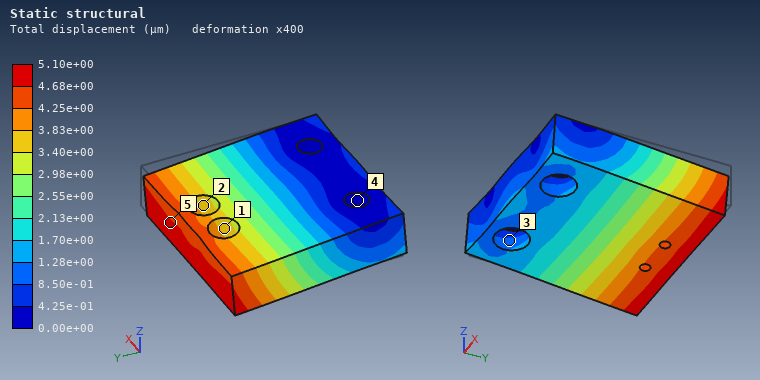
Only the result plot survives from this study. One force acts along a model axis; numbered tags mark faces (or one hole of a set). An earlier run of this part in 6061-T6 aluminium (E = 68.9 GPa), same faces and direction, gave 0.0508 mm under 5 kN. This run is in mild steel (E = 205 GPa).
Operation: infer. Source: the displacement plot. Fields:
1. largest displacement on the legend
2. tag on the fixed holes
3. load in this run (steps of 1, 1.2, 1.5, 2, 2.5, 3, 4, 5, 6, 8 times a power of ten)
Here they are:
5.10e+00 µm
4
1.5 kN
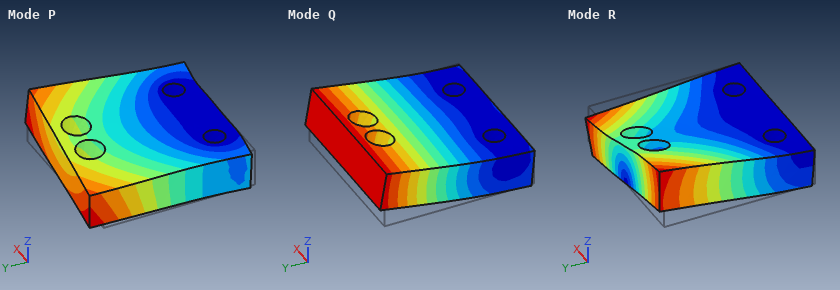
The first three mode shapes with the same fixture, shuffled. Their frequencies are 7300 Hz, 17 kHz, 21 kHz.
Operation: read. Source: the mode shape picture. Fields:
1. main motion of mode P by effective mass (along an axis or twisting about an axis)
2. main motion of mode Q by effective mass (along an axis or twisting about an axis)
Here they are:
along X
along Z
